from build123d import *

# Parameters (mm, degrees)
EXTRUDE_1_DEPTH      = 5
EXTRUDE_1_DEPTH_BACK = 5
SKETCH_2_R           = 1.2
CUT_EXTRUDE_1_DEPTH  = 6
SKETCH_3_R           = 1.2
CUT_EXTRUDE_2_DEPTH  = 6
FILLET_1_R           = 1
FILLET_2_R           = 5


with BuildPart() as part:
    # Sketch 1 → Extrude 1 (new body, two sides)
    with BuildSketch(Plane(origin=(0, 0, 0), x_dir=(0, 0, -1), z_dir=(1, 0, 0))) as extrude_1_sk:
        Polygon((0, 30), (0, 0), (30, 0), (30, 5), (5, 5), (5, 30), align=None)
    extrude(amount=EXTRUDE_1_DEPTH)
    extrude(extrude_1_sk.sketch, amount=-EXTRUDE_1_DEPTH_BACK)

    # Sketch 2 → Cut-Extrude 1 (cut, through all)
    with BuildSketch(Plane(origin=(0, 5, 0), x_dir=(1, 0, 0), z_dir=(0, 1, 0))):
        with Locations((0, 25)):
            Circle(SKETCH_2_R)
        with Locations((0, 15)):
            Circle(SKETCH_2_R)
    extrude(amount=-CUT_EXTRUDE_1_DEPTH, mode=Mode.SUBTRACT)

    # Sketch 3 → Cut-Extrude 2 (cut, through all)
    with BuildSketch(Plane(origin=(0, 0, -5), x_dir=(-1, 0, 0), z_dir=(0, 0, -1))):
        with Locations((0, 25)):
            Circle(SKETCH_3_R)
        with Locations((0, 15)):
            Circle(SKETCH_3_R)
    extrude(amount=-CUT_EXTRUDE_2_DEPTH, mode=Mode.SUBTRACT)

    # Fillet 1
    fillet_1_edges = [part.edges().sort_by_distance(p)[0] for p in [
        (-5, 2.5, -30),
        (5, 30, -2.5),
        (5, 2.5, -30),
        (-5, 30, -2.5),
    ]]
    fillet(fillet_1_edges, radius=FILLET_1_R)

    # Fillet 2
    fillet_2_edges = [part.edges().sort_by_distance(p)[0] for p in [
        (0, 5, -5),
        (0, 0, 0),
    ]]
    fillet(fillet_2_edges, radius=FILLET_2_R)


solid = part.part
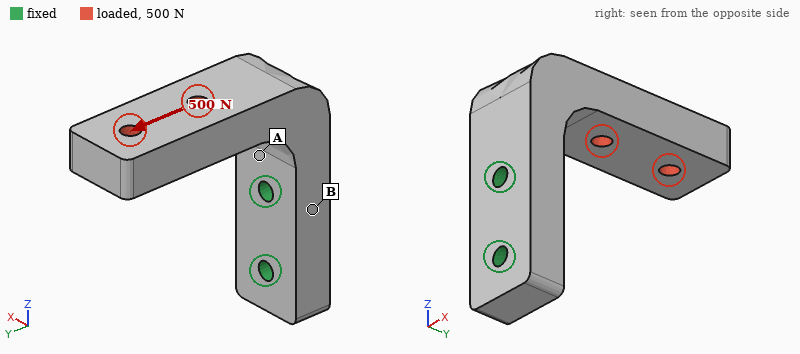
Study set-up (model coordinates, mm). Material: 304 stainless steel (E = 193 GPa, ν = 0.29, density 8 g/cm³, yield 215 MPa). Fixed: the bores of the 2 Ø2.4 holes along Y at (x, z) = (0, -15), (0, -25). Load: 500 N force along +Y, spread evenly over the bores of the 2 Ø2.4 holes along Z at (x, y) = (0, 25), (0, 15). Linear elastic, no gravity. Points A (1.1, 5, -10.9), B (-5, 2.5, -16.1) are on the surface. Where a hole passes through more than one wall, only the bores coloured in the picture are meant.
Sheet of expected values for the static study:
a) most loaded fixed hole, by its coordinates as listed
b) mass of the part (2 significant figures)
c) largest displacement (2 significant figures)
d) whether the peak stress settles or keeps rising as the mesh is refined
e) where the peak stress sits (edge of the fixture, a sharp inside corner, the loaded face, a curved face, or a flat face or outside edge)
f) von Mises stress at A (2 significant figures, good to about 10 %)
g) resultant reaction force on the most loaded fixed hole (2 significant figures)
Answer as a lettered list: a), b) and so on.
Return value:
a) (0, -15)
b) 21 g
c) 58 µm
d) keeps rising
e) edge of the fixture
f) 110 MPa
g) 650 N
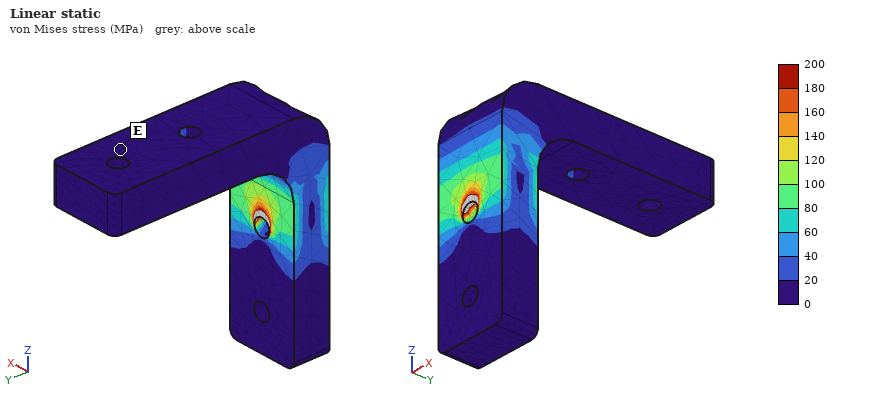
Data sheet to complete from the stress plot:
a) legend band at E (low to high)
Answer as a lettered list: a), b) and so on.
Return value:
a) 0 to 20 MPa
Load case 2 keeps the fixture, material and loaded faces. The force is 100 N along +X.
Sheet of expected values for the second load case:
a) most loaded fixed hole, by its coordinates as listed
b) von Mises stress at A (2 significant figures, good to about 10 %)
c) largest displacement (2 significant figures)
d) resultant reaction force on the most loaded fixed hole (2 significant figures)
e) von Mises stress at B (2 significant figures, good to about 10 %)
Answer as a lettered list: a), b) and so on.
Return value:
a) (0, -15)
b) 43 MPa
c) 25 µm
d) 180 N
e) 15 MPa
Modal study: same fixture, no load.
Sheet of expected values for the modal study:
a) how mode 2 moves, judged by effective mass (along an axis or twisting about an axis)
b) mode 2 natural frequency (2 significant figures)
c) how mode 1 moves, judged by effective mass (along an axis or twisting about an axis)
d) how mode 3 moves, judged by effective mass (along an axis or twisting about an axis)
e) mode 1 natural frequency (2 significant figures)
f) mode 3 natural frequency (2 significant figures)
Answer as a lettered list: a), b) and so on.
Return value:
a) along X
b) 4200 Hz
c) along Z
d) along Y
e) 3500 Hz
f) 12 kHz
